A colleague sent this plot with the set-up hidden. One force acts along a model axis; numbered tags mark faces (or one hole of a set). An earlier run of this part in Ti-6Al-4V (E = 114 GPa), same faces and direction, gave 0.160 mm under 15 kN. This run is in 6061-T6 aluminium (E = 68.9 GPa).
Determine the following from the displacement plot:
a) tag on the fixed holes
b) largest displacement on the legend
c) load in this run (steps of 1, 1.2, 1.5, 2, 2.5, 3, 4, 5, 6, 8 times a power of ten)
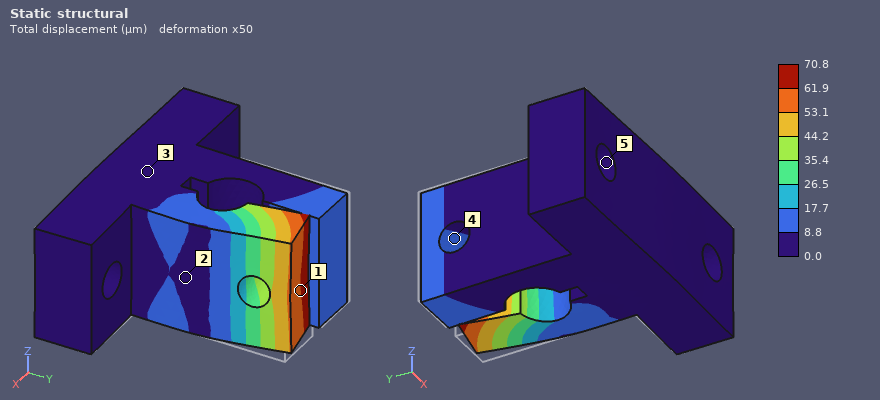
5
70.8 µm
4 kN
